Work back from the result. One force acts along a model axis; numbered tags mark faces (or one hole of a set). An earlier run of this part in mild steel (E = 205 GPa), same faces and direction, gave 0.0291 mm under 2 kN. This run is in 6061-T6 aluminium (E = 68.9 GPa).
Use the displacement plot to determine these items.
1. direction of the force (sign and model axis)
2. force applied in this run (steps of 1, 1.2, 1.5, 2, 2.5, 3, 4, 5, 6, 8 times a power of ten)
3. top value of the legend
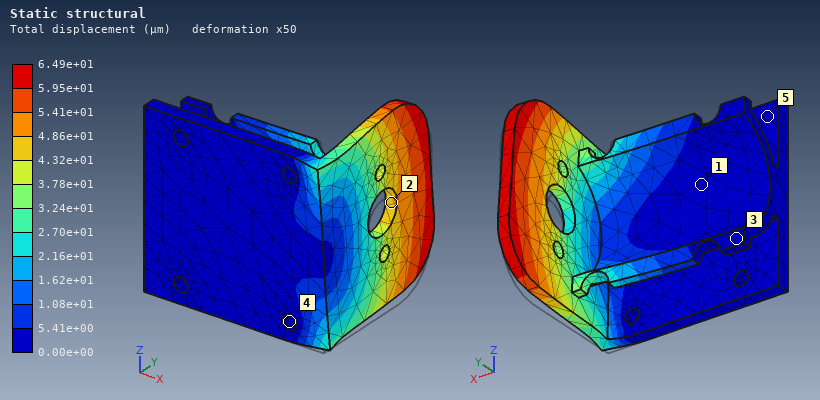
+Z
1.5 kN
6.49e+01 µm
